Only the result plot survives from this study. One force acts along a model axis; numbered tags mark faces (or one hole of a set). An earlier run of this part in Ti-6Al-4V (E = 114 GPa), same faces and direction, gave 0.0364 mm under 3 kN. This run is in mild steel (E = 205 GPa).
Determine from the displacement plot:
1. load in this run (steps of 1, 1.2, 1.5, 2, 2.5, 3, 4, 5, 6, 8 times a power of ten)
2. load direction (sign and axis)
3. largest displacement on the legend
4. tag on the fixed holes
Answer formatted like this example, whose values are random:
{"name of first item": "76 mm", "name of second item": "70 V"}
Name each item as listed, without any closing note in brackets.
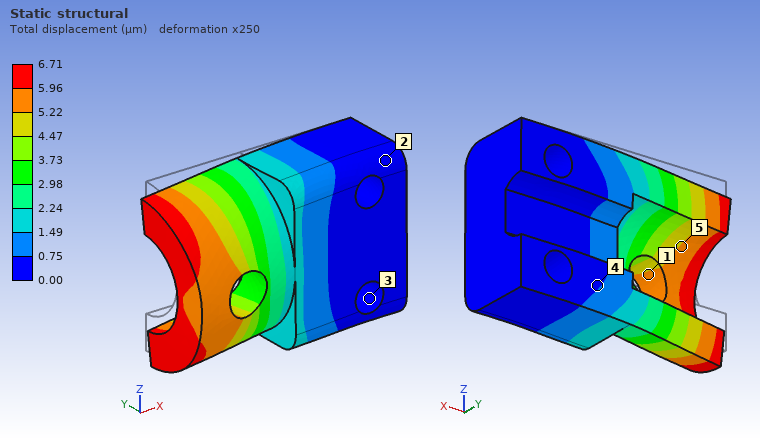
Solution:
{"load in this run": "1 kN", "load direction": "-Z", "largest displacement on the legend": "6.71 µm", "tag on the fixed holes": "3"}
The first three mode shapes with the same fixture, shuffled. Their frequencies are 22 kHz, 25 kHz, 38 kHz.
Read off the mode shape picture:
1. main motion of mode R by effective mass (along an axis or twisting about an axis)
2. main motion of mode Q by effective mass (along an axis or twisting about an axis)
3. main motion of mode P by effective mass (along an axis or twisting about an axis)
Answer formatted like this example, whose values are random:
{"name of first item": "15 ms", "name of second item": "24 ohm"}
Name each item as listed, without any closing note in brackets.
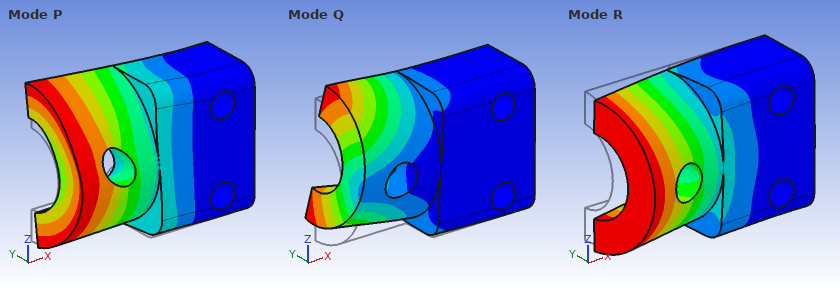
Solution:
{"main motion of mode R by effective mass": "along Y", "main motion of mode Q by effective mass": "along Z", "main motion of mode P by effective mass": "along Z"}
